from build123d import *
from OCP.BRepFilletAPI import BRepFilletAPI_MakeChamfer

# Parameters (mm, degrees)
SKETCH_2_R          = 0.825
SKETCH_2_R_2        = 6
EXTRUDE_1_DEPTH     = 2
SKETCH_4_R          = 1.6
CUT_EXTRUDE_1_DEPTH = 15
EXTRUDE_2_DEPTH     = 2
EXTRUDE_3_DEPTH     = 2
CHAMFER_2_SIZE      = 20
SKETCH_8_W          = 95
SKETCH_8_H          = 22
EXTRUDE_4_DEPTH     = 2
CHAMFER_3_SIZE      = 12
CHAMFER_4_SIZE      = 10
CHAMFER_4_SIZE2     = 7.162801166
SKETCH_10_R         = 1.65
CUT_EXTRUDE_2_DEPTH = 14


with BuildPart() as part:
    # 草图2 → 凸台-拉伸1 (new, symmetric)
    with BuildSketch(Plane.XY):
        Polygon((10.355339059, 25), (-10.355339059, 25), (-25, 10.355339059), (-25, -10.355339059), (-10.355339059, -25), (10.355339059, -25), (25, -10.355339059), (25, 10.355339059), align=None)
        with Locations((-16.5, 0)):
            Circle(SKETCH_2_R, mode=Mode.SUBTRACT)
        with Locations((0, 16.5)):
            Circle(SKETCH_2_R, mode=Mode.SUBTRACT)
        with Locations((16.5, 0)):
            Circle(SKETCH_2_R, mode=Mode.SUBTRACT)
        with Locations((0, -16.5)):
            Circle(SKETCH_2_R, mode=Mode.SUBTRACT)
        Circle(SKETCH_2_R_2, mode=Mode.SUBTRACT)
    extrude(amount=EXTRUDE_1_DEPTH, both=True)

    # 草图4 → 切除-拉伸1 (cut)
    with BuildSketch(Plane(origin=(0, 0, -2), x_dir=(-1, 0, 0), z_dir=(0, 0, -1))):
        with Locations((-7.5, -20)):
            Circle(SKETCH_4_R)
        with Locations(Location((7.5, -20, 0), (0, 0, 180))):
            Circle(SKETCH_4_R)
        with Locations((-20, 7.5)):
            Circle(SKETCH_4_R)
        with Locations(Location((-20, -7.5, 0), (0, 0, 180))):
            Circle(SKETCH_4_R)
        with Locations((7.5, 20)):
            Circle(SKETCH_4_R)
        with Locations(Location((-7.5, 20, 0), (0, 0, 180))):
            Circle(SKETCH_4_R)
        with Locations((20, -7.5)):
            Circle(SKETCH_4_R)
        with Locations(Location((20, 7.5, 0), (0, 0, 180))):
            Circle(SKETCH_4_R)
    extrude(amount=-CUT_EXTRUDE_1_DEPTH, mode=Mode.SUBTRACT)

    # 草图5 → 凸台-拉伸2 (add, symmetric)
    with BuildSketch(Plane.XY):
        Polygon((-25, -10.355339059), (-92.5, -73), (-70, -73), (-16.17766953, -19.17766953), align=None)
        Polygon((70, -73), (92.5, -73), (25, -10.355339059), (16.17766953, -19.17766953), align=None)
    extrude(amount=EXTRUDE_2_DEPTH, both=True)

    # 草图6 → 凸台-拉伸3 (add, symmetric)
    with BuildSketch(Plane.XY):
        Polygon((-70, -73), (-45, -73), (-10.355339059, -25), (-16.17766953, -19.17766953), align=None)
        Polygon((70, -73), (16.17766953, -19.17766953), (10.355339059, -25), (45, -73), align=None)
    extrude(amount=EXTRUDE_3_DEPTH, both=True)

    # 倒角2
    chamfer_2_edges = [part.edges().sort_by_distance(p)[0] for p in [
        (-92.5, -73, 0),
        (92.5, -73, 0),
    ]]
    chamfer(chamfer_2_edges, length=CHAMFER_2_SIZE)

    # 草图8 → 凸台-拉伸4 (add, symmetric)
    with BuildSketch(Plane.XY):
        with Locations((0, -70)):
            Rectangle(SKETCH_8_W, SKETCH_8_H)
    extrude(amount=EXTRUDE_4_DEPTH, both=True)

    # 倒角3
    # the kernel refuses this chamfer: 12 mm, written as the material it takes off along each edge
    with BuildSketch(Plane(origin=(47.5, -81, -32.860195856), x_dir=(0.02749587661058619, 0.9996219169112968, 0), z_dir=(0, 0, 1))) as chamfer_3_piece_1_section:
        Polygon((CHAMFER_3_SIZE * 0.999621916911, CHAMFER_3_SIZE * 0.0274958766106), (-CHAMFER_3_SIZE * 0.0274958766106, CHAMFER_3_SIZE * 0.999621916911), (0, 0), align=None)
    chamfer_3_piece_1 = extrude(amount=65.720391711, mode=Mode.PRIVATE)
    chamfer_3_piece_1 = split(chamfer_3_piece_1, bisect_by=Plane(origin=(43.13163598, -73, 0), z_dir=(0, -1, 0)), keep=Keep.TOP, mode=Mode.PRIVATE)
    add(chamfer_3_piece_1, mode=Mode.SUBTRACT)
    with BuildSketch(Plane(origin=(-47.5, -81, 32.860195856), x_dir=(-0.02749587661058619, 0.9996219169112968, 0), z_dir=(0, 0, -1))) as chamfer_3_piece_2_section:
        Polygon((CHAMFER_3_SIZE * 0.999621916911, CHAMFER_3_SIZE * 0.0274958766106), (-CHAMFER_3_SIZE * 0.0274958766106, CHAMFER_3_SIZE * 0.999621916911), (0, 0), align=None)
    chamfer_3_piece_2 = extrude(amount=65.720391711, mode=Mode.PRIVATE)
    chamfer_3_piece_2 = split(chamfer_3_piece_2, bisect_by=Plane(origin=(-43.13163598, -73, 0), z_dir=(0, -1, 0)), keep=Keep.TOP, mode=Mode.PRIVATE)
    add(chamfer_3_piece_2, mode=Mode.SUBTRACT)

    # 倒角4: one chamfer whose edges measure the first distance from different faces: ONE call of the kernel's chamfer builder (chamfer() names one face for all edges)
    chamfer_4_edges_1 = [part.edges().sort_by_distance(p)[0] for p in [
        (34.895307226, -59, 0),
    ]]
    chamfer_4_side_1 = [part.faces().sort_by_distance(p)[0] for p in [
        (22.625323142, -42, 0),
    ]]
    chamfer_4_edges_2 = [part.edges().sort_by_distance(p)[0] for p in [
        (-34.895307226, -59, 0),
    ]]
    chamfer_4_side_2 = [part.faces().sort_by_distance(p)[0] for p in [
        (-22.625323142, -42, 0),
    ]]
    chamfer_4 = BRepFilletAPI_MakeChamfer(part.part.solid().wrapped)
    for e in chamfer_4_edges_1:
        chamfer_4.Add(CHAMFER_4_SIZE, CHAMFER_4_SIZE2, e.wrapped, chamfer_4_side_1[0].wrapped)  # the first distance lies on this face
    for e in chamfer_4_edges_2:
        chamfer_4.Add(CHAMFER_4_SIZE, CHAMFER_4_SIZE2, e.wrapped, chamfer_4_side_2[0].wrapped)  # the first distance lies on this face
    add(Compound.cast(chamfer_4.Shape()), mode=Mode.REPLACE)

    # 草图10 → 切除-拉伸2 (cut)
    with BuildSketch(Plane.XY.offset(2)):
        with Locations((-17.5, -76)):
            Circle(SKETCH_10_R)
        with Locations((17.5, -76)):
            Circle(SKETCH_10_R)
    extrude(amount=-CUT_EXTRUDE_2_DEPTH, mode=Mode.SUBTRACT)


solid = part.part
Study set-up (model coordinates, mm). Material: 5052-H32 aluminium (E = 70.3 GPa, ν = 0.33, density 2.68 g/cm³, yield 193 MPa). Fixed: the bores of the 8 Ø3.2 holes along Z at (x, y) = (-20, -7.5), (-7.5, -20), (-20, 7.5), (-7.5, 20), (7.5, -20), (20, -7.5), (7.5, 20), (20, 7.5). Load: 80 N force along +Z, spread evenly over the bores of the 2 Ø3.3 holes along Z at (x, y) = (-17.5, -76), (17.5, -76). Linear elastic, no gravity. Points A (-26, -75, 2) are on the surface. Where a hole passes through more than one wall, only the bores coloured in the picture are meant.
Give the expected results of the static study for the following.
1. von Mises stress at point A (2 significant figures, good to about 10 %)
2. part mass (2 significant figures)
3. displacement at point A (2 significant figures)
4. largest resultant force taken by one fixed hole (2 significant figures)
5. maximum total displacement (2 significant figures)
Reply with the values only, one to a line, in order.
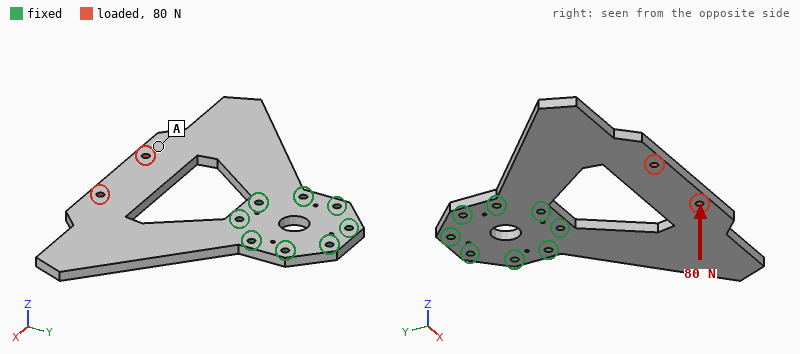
5.6 MPa
81 g
0.39 mm
110 N
0.45 mm
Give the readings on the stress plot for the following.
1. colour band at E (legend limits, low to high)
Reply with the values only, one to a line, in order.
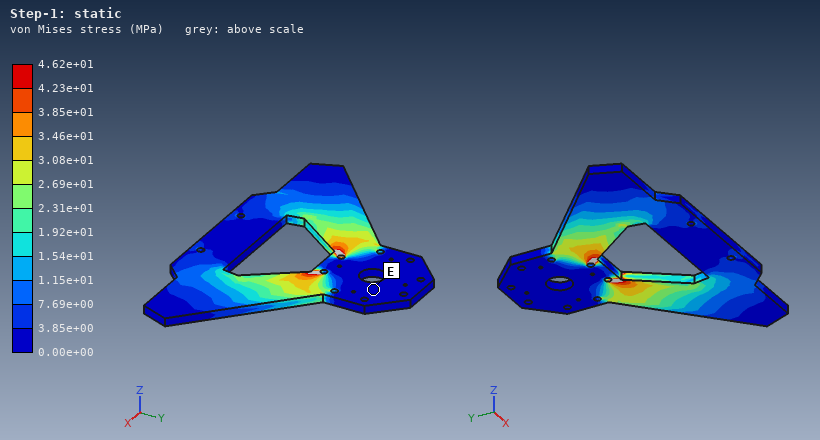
0.00e+00 to 3.85e+00 MPa
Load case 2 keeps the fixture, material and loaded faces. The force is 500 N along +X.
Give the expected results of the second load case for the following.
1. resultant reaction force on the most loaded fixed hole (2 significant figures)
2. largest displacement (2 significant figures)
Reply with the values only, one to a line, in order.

660 N
71 µm
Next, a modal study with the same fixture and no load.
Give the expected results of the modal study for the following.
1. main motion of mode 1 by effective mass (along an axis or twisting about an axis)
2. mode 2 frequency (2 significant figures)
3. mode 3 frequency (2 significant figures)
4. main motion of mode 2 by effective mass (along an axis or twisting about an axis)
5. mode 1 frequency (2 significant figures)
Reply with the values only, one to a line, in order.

along Z
520 Hz
1200 Hz
twisting about Y
420 Hz
